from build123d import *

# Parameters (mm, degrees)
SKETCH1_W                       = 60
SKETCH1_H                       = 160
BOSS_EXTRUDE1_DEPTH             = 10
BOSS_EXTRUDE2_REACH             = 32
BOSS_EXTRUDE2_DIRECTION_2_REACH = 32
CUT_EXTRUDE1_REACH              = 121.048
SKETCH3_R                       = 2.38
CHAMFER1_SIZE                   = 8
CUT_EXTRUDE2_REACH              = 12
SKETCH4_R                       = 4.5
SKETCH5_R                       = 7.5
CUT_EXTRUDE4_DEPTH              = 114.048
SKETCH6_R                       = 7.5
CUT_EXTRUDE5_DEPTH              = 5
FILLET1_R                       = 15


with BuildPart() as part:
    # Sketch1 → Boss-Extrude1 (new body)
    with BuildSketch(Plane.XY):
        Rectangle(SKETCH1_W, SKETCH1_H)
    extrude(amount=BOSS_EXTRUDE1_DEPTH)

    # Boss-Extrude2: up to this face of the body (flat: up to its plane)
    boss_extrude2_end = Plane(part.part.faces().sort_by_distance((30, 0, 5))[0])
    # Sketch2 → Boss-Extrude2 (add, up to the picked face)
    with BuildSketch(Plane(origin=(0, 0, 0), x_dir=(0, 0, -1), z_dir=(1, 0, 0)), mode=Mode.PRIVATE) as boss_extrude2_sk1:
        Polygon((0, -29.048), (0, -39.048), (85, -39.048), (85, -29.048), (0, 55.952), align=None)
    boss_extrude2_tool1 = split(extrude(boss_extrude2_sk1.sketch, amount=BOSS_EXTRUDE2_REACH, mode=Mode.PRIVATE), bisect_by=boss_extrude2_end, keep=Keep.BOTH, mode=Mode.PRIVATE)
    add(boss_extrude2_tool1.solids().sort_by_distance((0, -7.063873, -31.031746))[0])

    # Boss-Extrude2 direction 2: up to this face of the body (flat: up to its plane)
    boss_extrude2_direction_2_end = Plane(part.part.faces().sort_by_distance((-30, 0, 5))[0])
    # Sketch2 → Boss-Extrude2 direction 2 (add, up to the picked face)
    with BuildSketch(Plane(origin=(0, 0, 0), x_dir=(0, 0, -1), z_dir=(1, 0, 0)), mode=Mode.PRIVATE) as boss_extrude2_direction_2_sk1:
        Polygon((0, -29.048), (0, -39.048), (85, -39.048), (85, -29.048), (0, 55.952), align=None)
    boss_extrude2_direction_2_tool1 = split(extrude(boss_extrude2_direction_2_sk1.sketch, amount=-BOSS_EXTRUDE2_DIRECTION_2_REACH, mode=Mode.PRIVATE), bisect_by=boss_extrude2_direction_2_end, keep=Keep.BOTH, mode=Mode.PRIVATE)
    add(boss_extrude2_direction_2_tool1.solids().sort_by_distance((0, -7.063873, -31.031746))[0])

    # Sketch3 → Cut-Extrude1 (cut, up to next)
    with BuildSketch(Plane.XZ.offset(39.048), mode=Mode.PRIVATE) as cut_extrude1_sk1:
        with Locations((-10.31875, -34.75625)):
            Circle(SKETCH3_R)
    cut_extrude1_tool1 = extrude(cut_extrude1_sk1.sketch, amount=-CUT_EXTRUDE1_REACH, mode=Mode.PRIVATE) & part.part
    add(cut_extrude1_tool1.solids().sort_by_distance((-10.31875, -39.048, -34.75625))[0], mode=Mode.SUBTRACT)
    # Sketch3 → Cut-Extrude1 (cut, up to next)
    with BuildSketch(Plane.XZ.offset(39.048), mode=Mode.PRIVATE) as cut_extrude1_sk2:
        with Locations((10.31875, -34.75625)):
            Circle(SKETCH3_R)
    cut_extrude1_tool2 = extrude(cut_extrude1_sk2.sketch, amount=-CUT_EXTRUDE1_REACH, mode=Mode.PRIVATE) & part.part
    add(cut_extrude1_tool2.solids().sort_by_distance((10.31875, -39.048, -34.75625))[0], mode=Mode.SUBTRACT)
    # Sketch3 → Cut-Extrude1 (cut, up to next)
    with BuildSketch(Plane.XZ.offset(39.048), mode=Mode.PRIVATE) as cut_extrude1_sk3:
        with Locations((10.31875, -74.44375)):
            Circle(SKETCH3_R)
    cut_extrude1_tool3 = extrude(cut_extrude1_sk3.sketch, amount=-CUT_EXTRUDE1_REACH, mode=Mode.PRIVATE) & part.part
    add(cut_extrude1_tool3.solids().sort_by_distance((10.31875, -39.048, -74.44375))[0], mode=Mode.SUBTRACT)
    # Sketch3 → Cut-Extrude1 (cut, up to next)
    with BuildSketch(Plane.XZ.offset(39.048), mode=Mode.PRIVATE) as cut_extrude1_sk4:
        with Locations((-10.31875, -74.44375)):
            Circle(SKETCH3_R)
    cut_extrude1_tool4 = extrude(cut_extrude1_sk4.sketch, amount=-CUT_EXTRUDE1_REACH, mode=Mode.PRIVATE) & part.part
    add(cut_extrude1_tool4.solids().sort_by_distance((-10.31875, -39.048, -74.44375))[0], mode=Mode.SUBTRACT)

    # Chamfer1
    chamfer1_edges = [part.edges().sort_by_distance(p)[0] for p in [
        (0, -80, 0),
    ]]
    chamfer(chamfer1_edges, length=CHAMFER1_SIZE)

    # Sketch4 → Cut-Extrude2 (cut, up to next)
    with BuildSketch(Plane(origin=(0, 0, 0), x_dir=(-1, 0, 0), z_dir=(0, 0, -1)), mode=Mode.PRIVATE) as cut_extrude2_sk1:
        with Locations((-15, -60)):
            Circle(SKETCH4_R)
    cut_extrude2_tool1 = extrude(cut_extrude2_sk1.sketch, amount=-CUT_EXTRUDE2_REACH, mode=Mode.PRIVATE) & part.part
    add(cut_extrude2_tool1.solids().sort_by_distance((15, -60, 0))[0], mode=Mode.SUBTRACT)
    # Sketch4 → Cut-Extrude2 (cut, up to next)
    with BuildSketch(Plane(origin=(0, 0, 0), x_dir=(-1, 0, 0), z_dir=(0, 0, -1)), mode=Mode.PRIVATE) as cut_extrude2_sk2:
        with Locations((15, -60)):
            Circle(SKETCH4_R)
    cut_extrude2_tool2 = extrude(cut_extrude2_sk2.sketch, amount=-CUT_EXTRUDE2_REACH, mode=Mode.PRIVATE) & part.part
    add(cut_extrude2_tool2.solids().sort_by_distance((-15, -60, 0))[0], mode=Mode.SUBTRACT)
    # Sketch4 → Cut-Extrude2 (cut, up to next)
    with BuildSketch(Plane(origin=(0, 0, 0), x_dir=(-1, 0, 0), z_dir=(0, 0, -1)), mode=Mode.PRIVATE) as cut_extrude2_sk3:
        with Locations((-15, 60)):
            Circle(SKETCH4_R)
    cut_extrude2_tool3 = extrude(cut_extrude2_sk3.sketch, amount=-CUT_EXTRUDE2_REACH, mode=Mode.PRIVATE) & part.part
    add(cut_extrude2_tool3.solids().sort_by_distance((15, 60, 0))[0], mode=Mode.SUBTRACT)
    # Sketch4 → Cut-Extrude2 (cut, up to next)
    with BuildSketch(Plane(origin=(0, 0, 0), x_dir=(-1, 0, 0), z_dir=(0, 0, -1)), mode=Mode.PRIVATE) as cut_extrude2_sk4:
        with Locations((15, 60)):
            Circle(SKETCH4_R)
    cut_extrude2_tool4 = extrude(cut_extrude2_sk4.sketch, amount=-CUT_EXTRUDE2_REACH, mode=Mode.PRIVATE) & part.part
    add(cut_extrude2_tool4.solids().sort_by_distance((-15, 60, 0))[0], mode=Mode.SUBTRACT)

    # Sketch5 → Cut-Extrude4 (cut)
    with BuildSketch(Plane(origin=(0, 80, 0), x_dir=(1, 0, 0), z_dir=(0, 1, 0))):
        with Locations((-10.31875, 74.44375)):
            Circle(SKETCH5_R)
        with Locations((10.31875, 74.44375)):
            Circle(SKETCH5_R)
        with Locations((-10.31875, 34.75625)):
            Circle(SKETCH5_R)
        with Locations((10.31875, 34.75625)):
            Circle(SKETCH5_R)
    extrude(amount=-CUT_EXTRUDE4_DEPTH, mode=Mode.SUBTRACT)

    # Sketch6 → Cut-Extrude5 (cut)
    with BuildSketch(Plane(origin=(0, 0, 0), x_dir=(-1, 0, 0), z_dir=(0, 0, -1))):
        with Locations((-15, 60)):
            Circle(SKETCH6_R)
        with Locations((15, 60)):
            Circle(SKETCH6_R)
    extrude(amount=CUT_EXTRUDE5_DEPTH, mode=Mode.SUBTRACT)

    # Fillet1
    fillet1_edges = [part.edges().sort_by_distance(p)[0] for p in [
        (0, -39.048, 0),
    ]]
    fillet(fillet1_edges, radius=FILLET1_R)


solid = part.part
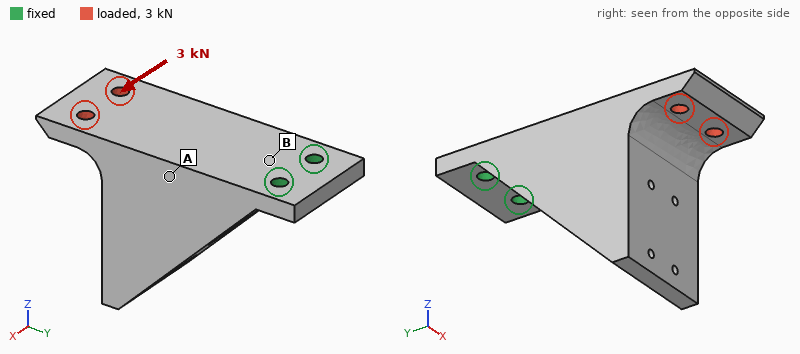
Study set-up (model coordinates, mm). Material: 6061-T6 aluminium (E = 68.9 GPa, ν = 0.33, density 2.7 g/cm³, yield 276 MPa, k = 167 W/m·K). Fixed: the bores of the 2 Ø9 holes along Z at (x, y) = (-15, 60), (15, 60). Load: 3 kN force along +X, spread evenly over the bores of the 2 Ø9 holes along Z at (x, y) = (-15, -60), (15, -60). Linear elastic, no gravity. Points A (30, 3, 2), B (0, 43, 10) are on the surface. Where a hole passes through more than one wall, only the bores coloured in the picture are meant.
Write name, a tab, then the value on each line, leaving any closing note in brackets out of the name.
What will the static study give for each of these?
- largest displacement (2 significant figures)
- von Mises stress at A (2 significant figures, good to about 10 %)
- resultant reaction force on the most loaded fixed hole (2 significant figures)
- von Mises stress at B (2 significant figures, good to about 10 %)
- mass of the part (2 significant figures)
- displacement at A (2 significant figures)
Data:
largest displacement	0.16 mm
von Mises stress at A	11 MPa
resultant reaction force on the most loaded fixed hole	10 kN
von Mises stress at B	30 MPa
mass of the part	910 g
displacement at A	0.061 mm
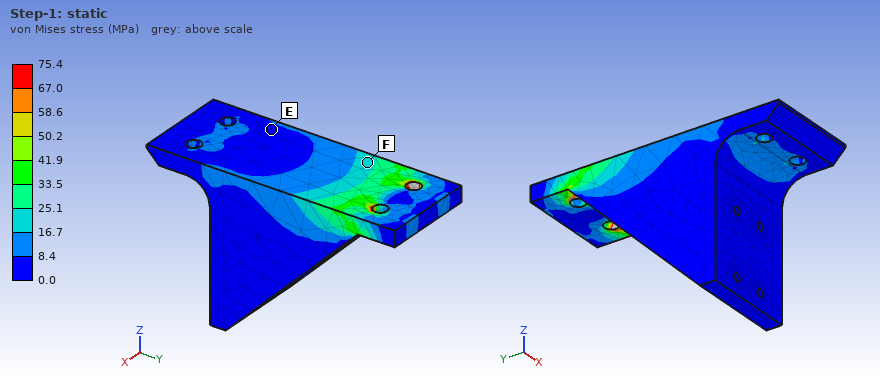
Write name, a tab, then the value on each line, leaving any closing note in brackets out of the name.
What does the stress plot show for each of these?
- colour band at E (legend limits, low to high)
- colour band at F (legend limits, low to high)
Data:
colour band at E	0.0 to 8.4 MPa
colour band at F	16.7 to 25.1 MPa
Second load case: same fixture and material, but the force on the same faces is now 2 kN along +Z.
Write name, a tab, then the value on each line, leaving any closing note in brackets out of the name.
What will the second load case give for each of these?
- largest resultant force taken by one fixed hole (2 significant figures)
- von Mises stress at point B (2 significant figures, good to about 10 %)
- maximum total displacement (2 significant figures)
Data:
largest resultant force taken by one fixed hole	1.0 kN
von Mises stress at point B	59 MPa
maximum total displacement	0.98 mm
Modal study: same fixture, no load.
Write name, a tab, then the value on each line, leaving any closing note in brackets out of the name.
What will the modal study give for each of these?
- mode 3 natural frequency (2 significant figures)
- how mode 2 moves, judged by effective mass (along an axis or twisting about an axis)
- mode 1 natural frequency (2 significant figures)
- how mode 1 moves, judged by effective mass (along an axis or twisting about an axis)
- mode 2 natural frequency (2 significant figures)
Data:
mode 3 natural frequency	2000 Hz
how mode 2 moves, judged by effective mass	along X
mode 1 natural frequency	410 Hz
how mode 1 moves, judged by effective mass	along Z
mode 2 natural frequency	1400 Hz
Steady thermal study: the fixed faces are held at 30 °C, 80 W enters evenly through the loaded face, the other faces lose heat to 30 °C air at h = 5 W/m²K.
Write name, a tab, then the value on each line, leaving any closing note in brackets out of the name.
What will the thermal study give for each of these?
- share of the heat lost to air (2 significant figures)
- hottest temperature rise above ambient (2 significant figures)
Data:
share of the heat lost to air	6.0 %
hottest temperature rise above ambient	50 K
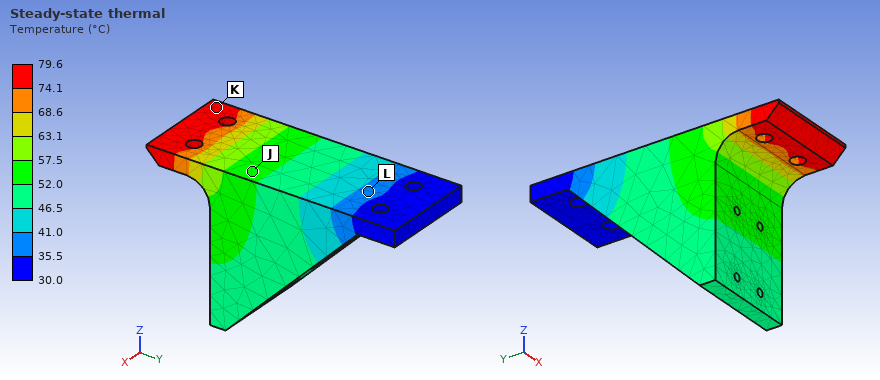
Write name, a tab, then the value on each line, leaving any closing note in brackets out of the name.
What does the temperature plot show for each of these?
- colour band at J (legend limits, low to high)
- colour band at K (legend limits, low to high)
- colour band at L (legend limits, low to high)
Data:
colour band at J	52.0 to 57.5 °C
colour band at K	74.1 to 79.6 °C
colour band at L	35.5 to 41.0 °C
